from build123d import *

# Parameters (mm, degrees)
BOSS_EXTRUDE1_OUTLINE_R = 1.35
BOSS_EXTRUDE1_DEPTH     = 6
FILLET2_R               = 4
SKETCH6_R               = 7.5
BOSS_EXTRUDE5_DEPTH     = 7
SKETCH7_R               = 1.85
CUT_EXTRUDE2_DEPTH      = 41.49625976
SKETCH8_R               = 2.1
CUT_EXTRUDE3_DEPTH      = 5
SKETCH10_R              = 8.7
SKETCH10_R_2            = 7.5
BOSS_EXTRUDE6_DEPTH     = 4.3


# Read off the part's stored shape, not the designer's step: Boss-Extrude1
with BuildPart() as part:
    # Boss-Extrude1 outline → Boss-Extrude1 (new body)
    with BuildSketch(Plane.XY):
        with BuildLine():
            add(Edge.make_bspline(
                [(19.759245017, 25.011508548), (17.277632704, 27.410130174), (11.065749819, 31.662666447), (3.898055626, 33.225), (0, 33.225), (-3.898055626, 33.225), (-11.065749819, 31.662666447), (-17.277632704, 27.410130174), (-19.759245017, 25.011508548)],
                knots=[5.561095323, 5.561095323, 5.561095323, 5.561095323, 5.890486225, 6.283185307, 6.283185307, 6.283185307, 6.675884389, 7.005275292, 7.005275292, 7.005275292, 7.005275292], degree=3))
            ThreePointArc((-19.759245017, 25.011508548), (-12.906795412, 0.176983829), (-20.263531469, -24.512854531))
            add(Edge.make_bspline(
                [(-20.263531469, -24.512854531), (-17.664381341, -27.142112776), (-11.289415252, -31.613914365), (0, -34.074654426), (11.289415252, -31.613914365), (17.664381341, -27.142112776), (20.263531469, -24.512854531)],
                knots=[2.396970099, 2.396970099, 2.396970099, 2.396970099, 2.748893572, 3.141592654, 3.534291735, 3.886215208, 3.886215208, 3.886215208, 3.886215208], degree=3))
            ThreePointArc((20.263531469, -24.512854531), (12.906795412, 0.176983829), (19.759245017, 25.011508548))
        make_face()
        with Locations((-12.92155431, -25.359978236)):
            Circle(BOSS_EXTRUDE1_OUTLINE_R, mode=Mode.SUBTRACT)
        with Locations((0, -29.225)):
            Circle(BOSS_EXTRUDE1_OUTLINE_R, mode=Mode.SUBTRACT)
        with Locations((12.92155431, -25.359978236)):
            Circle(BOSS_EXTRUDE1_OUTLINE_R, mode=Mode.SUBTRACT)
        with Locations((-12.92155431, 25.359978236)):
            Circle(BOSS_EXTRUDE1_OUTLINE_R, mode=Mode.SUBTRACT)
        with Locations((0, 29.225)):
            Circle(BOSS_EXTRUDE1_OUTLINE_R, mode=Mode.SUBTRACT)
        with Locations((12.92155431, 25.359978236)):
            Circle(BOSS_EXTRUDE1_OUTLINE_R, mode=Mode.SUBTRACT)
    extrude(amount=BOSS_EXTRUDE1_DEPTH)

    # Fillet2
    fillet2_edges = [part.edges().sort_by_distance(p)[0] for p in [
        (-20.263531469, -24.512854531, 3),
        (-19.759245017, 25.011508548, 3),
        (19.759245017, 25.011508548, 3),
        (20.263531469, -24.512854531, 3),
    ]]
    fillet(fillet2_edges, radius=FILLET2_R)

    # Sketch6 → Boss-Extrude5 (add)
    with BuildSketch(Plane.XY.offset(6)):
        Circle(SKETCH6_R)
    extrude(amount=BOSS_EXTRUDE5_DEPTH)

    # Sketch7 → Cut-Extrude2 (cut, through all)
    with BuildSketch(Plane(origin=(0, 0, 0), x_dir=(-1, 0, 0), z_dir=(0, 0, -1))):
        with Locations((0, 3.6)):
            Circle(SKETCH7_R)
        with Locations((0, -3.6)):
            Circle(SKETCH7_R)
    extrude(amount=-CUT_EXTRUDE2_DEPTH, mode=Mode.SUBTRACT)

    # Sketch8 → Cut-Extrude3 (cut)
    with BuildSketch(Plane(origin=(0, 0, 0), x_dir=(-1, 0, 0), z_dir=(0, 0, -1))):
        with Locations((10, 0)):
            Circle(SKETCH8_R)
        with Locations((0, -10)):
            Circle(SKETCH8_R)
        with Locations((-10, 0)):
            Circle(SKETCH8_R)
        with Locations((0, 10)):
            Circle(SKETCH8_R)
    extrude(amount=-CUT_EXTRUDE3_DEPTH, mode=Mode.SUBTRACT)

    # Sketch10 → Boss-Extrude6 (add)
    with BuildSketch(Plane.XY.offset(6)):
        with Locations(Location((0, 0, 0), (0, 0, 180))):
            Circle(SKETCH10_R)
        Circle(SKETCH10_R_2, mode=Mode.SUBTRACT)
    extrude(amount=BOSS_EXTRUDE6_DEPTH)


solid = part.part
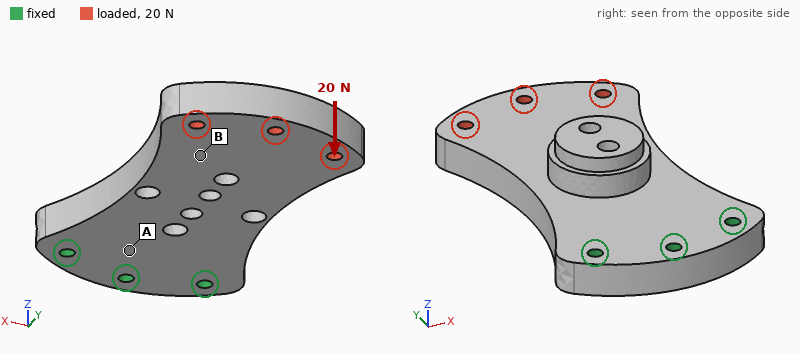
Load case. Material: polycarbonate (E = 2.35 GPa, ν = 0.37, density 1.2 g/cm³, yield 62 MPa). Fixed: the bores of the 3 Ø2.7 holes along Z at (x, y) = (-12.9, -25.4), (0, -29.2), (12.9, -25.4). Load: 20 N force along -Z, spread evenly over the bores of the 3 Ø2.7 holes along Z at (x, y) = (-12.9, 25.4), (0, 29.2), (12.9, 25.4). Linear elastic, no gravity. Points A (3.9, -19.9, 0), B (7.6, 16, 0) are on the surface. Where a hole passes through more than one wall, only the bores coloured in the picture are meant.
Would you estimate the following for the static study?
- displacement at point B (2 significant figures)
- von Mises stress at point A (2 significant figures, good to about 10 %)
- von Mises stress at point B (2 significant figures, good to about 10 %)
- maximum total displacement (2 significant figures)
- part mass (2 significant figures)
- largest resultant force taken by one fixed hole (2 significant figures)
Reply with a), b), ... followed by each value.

a) 0.52 mm
b) 3.7 MPa
c) 1.1 MPa
d) 0.86 mm
e) 15 g
f) 15 N
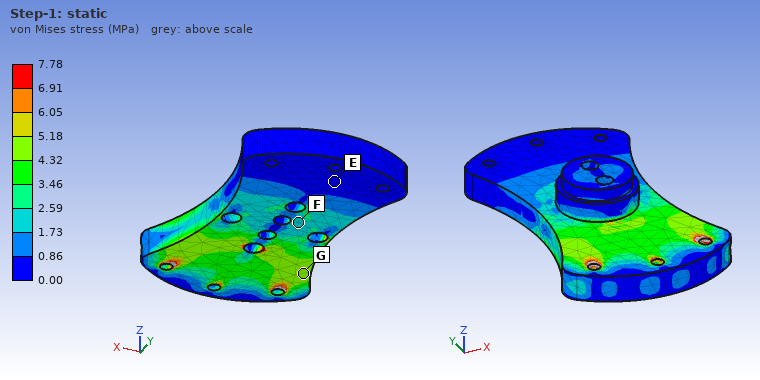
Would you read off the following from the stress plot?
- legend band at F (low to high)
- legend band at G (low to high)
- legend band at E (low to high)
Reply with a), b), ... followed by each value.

a) 1.73 to 2.59 MPa
b) 4.32 to 5.18 MPa
c) 0.00 to 0.86 MPa
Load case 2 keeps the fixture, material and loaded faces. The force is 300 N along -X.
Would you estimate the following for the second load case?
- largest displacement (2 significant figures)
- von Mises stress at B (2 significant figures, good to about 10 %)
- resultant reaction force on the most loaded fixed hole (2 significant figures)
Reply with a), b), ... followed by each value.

a) 0.77 mm
b) 4.1 MPa
c) 600 N
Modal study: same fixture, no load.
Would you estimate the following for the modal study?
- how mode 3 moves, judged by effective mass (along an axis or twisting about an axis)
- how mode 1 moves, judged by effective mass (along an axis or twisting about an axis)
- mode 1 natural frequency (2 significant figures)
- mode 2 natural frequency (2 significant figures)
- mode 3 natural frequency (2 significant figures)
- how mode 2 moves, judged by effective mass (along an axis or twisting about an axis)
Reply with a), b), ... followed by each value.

a) along X
b) along Z
c) 400 Hz
d) 1500 Hz
e) 1600 Hz
f) along X
